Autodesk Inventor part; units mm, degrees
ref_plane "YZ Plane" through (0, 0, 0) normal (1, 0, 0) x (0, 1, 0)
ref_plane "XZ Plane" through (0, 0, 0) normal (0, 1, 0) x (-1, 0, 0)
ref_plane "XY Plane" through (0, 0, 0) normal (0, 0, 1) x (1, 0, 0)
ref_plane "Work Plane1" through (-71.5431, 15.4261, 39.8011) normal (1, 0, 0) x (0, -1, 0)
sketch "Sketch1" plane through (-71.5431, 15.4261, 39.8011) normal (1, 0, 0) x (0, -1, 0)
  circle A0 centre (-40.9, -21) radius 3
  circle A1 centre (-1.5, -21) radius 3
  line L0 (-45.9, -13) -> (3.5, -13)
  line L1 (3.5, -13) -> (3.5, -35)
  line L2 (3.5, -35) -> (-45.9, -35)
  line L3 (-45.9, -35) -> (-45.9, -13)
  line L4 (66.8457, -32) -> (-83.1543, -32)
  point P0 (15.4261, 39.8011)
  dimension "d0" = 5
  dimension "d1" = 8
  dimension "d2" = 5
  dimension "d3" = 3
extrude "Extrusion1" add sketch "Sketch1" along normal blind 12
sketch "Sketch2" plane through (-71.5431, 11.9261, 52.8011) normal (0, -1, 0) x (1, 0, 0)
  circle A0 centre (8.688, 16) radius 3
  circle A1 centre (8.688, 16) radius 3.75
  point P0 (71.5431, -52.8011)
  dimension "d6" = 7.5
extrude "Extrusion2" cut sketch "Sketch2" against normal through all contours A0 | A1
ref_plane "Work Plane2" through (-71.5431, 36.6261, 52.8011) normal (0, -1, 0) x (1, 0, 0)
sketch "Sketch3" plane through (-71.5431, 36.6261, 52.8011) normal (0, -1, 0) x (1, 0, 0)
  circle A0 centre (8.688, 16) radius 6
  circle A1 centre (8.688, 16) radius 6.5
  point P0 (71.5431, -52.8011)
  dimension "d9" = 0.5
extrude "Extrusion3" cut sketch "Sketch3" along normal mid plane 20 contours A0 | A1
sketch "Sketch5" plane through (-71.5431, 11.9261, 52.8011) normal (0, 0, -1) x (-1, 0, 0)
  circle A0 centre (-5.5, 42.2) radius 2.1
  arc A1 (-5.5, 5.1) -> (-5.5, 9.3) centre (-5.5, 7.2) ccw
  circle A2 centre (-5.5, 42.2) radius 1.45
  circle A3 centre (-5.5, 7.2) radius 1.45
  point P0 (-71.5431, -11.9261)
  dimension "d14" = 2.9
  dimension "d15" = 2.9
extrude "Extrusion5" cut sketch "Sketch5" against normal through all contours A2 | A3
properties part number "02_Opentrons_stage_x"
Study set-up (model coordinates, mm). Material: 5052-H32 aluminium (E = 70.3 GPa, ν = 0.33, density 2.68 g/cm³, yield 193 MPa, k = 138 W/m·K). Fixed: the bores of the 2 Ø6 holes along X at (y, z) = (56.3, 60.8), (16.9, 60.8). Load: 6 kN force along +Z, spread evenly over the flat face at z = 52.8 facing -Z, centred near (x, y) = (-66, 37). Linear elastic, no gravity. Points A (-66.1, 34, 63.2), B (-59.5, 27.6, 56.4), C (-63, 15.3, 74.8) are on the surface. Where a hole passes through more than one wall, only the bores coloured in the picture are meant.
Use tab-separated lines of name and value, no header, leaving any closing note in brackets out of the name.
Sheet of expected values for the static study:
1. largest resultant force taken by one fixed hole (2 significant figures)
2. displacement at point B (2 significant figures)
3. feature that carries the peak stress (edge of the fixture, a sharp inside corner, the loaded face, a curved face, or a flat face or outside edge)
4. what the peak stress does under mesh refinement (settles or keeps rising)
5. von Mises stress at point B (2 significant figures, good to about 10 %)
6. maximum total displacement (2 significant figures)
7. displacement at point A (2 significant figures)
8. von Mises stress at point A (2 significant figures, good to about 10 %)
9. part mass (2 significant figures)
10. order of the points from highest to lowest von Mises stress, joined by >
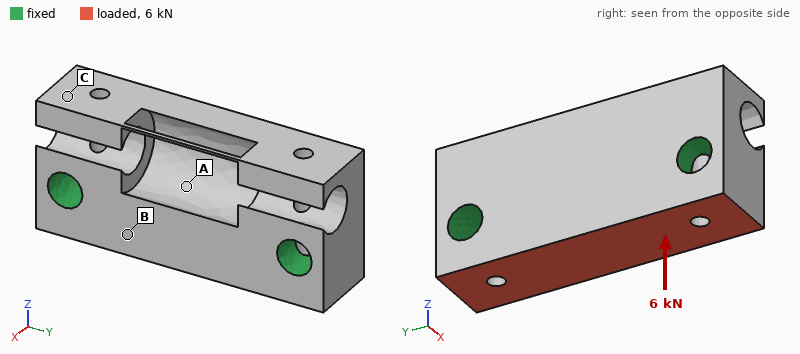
largest resultant force taken by one fixed hole	3.0 kN
displacement at point B	8.2 µm
feature that carries the peak stress	edge of the fixture
what the peak stress does under mesh refinement	keeps rising
von Mises stress at point B	22 MPa
maximum total displacement	13 µm
displacement at point A	9.6 µm
von Mises stress at point A	15 MPa
part mass	24 g
order of the points from highest to lowest von Mises stress, joined by >	B > A > C
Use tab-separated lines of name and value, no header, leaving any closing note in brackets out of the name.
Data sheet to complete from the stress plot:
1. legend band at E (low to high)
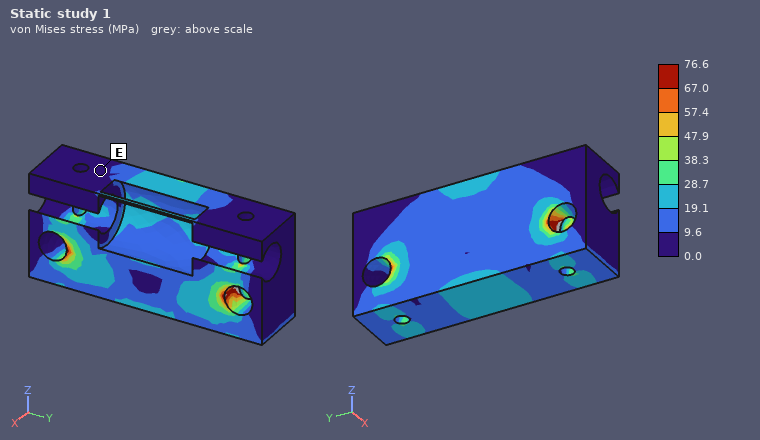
legend band at E	0.0 to 9.6 MPa
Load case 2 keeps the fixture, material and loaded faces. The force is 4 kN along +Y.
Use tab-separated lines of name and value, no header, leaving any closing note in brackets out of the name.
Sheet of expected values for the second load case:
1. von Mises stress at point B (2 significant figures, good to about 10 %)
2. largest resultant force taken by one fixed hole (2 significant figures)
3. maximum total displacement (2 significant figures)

von Mises stress at point B	12 MPa
largest resultant force taken by one fixed hole	2.1 kN
maximum total displacement	3.9 µm
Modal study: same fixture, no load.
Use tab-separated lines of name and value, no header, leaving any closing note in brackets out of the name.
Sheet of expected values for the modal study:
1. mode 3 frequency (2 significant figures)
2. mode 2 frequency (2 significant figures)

mode 3 frequency	11 kHz
mode 2 frequency	8700 Hz
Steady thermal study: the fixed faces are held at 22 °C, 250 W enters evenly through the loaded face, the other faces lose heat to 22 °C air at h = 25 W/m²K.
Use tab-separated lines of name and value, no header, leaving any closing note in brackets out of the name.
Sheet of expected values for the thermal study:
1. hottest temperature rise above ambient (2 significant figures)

hottest temperature rise above ambient	58 K
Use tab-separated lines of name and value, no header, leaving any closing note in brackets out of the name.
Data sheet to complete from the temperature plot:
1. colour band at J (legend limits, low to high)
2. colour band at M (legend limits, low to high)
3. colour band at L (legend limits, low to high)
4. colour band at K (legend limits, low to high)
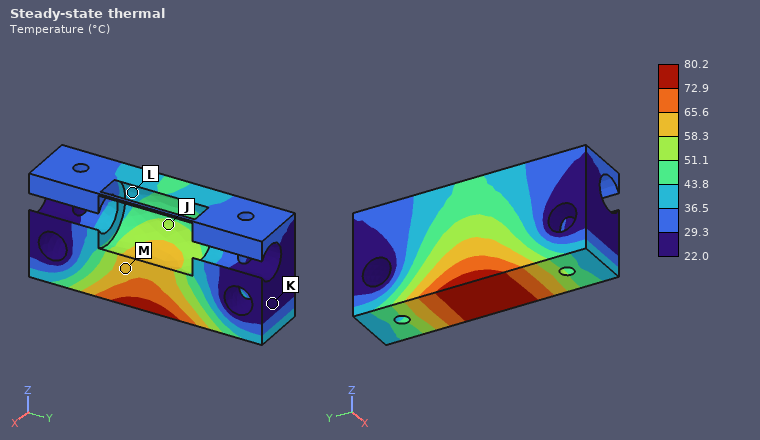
colour band at J	51.1 to 58.3 °C
colour band at M	58.3 to 65.6 °C
colour band at L	36.5 to 43.8 °C
colour band at K	22.0 to 29.3 °C
